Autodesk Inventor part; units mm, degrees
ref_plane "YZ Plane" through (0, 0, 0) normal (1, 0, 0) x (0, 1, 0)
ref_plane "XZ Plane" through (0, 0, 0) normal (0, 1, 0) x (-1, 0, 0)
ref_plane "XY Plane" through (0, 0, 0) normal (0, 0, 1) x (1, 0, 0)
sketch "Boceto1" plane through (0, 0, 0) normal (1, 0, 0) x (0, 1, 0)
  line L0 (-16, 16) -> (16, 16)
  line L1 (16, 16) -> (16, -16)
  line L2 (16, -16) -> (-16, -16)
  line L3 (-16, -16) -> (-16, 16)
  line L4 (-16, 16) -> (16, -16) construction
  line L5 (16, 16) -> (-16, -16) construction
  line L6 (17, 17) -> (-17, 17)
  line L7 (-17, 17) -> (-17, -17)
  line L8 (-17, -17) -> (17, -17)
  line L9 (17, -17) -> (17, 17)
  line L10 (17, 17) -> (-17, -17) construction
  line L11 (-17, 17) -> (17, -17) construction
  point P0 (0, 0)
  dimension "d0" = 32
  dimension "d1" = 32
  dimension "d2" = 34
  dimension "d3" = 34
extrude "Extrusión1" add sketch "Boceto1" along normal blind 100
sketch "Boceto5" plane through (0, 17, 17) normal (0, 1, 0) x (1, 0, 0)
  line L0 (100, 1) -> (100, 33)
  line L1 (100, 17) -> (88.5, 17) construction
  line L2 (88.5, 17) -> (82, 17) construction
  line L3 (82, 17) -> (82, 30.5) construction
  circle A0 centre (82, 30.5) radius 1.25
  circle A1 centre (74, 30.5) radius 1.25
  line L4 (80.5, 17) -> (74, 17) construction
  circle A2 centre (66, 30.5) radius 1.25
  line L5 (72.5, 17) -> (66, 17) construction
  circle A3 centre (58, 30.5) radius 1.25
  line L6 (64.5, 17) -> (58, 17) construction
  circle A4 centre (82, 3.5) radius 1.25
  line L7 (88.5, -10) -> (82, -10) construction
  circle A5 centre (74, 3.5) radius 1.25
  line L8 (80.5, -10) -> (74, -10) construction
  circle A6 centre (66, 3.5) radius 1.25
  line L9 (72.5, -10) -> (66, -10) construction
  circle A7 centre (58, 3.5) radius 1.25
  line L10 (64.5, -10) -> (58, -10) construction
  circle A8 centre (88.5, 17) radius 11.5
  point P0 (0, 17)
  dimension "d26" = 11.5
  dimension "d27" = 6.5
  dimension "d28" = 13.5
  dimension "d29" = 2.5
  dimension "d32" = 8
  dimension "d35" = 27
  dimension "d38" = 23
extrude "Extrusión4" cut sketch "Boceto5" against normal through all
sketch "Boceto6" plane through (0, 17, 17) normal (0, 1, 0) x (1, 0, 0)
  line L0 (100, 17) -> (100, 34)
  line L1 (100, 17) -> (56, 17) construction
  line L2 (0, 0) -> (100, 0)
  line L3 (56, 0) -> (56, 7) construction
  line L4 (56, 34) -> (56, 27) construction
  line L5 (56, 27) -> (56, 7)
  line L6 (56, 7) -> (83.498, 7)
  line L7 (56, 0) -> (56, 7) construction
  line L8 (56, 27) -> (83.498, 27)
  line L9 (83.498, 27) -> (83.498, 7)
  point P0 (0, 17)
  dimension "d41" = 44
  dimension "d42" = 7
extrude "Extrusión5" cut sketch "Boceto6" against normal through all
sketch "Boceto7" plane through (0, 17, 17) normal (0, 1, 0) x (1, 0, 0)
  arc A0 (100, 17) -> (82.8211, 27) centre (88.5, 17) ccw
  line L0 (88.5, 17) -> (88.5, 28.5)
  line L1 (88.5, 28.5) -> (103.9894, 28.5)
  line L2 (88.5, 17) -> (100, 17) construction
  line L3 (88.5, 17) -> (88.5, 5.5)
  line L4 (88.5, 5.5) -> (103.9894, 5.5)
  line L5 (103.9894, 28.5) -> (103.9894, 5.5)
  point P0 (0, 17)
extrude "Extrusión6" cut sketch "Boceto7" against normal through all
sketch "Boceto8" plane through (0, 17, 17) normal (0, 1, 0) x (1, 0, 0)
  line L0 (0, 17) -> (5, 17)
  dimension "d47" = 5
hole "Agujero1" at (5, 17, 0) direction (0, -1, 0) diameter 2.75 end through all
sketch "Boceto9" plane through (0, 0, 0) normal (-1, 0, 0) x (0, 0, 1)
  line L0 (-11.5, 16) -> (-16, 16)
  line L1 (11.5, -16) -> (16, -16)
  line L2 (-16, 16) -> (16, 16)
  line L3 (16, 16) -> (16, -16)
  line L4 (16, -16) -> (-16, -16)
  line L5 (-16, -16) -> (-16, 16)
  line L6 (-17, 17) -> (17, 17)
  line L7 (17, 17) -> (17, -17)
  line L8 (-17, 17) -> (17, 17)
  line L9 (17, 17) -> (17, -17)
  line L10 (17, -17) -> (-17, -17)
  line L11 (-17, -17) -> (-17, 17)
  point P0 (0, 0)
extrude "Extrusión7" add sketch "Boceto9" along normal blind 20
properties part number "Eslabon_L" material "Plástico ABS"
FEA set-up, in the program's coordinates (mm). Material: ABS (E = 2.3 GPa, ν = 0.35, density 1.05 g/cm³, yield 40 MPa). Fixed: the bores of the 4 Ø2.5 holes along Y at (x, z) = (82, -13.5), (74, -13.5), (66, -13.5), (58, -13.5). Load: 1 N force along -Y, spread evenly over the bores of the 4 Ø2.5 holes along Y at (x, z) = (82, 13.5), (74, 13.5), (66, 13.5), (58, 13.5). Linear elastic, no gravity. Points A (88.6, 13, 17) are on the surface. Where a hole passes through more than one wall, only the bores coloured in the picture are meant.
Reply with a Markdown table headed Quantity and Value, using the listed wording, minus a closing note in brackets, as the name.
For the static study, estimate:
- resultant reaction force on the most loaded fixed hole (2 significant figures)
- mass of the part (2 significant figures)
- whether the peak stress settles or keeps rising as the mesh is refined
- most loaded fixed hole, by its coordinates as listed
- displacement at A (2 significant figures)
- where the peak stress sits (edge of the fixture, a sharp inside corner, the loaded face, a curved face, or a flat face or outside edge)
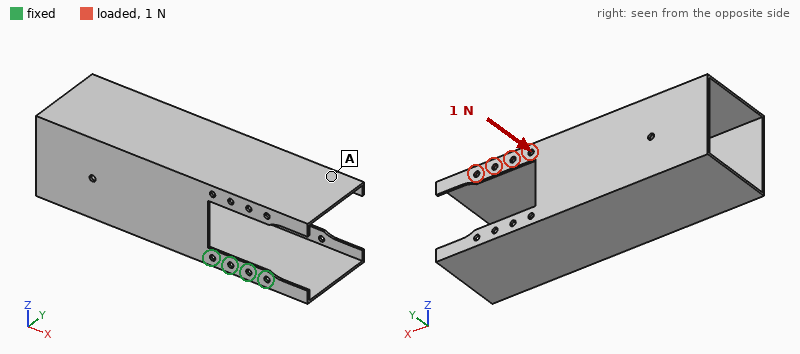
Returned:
| Quantity | Value |
|---|---|
| resultant reaction force on the most loaded fixed hole | 1.3 N |
| mass of the part | 15 g |
| whether the peak stress settles or keeps rising as the mesh is refined | keeps rising |
| most loaded fixed hole, by its coordinates as listed | (82, -13.5) |
| displacement at A | 1.5 mm |
| where the peak stress sits | edge of the fixture |
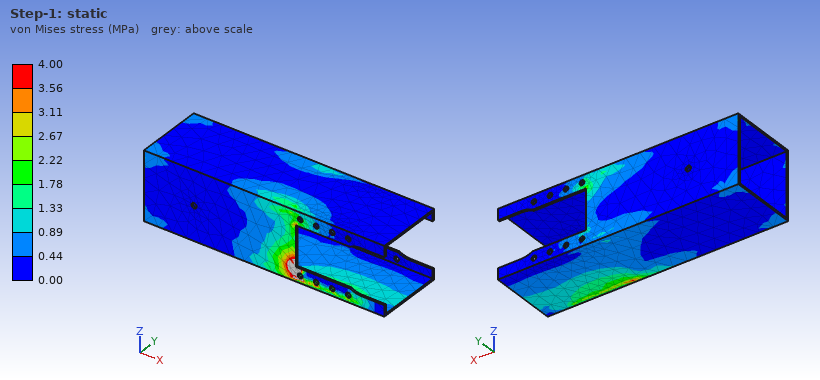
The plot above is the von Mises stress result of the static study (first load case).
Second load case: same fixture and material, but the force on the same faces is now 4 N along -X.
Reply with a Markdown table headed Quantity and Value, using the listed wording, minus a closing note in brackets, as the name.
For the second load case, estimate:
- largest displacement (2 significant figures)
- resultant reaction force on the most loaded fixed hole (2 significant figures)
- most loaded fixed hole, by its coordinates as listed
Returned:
| Quantity | Value |
|---|---|
| largest displacement | 1.3 mm |
| resultant reaction force on the most loaded fixed hole | 11 N |
| most loaded fixed hole, by its coordinates as listed | (58, -13.5) |
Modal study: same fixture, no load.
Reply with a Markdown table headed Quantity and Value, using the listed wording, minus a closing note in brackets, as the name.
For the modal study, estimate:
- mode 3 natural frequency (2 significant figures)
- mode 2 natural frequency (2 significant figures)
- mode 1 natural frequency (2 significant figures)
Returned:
| Quantity | Value |
|---|---|
| mode 3 natural frequency | 160 Hz |
| mode 2 natural frequency | 110 Hz |
| mode 1 natural frequency | 45 Hz |
